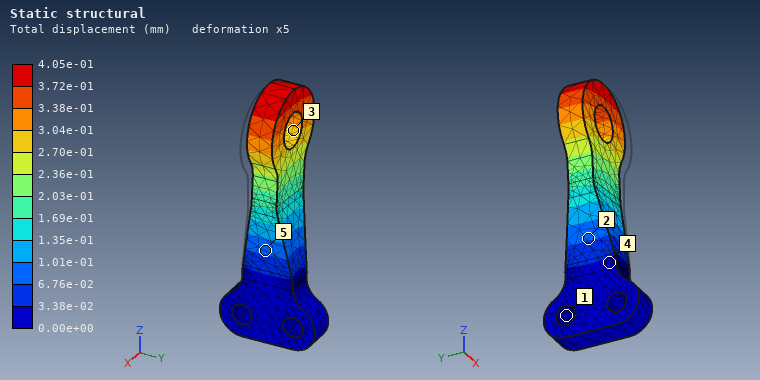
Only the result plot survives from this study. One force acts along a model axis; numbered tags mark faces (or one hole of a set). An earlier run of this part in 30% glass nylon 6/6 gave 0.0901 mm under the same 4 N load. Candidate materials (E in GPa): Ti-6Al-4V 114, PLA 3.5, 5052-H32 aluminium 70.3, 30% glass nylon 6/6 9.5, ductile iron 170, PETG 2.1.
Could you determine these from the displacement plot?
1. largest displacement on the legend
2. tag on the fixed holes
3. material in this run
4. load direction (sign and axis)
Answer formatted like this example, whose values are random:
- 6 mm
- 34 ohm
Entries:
- 4.05e-01 mm
- 1
- PETG
- -X
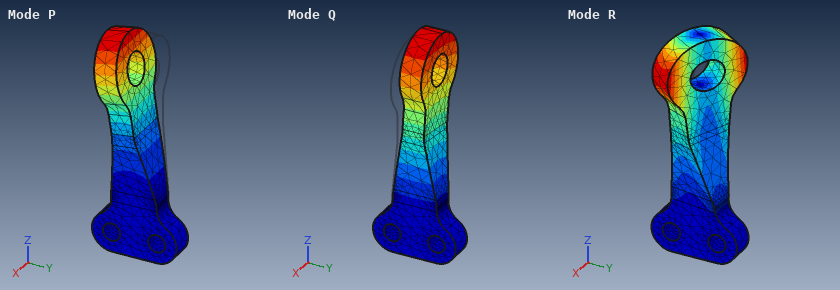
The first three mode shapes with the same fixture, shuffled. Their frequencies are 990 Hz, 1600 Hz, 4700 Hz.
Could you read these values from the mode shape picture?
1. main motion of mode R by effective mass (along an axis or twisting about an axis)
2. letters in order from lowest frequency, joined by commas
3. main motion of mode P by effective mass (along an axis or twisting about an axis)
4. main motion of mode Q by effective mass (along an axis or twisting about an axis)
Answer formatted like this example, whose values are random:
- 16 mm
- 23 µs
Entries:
- twisting about Z
- Q, P, R
- along Y
- along X
